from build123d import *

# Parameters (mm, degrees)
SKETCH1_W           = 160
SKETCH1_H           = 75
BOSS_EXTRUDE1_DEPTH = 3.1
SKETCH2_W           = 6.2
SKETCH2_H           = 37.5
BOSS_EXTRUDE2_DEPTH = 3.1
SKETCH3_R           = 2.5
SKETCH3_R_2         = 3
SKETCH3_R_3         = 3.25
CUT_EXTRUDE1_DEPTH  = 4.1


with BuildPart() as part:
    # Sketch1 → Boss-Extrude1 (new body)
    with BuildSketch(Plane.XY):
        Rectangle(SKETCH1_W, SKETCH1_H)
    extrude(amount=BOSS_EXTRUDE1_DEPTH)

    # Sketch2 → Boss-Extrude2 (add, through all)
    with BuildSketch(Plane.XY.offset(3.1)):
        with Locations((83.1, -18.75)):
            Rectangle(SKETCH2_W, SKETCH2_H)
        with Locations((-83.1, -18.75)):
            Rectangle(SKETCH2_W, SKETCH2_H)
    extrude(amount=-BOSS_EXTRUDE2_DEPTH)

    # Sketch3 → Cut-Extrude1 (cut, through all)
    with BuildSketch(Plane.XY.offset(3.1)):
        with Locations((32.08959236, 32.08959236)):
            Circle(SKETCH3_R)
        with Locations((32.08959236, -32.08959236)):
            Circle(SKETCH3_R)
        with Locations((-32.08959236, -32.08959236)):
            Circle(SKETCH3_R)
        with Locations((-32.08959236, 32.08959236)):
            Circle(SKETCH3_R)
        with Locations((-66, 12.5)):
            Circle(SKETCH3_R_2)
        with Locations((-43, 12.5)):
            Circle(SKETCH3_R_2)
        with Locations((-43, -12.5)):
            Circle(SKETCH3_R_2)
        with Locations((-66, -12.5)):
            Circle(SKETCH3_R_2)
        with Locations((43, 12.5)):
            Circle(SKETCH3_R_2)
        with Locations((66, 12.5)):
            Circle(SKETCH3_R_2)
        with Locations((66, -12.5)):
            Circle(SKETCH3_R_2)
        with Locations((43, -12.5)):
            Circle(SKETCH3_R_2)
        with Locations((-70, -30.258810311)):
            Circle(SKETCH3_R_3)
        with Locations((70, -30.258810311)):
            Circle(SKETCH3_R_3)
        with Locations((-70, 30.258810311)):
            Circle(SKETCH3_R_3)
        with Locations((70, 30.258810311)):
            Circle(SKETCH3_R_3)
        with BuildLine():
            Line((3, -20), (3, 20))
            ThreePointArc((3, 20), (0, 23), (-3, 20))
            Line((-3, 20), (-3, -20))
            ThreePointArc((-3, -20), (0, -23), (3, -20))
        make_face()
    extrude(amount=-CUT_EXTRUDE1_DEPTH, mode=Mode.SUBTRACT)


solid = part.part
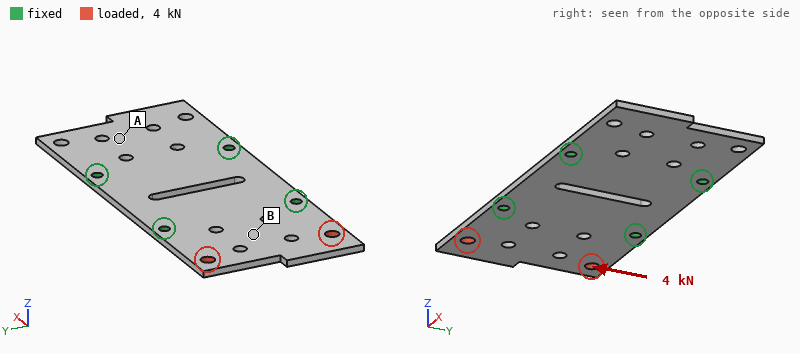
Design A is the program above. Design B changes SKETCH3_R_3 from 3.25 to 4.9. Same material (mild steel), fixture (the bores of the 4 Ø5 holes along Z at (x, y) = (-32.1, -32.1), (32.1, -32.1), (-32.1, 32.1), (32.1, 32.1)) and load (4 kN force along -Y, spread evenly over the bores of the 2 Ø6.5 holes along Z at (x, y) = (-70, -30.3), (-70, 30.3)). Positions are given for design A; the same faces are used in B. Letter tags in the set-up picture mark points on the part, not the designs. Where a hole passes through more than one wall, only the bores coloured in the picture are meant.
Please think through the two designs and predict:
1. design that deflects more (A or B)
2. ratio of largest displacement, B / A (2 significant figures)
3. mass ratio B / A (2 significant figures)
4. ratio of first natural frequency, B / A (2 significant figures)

B
1.1
0.99
1.0
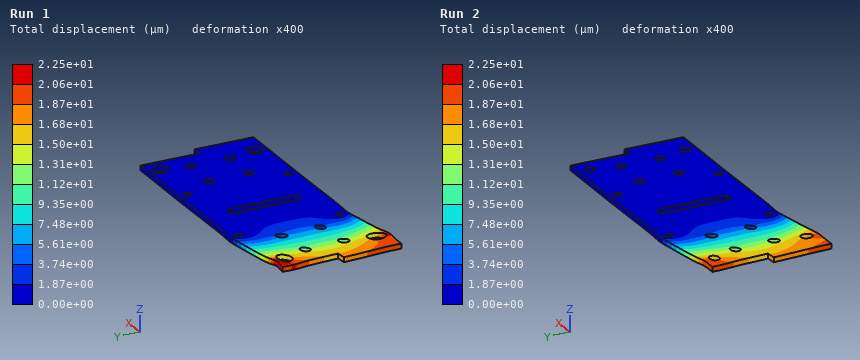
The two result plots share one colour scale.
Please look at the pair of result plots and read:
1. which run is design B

Run 1
